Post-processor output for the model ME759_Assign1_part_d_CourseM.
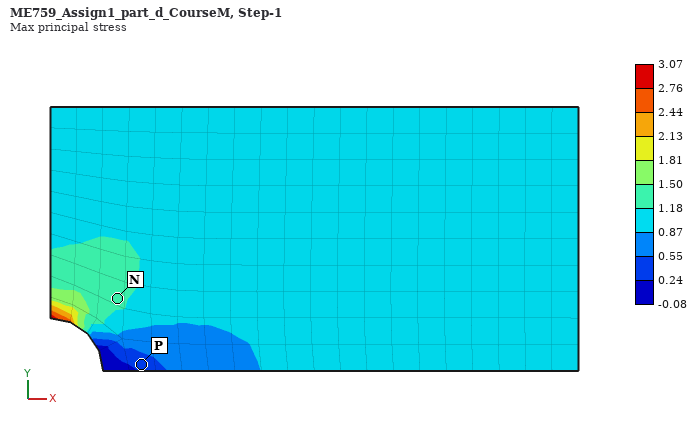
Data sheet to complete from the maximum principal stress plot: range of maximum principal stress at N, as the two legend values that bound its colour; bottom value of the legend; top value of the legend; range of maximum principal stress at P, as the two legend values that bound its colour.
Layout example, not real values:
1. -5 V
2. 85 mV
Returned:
1. 1.18 to 1.50
2. -0.08
3. 3.07
4. 0.24 to 0.55
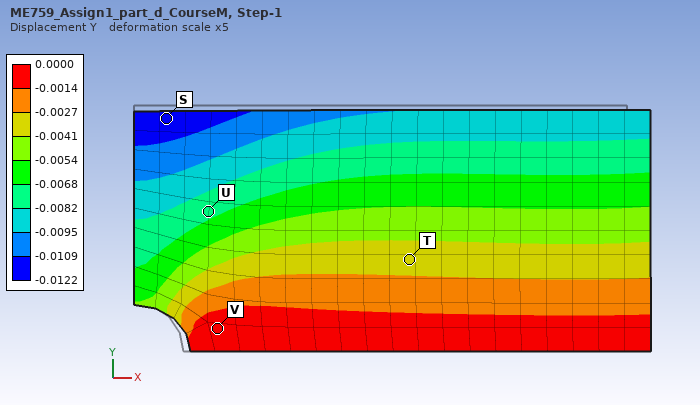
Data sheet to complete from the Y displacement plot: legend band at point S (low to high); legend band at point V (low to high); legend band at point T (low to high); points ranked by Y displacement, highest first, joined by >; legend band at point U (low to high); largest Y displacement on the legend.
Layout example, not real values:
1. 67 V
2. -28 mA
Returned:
1. -0.0122 to -0.0109
2. -0.0014 to 0.0000
3. -0.0041 to -0.0027
4. V > T > U > S
5. -0.0082 to -0.0068
6. 0.0000
